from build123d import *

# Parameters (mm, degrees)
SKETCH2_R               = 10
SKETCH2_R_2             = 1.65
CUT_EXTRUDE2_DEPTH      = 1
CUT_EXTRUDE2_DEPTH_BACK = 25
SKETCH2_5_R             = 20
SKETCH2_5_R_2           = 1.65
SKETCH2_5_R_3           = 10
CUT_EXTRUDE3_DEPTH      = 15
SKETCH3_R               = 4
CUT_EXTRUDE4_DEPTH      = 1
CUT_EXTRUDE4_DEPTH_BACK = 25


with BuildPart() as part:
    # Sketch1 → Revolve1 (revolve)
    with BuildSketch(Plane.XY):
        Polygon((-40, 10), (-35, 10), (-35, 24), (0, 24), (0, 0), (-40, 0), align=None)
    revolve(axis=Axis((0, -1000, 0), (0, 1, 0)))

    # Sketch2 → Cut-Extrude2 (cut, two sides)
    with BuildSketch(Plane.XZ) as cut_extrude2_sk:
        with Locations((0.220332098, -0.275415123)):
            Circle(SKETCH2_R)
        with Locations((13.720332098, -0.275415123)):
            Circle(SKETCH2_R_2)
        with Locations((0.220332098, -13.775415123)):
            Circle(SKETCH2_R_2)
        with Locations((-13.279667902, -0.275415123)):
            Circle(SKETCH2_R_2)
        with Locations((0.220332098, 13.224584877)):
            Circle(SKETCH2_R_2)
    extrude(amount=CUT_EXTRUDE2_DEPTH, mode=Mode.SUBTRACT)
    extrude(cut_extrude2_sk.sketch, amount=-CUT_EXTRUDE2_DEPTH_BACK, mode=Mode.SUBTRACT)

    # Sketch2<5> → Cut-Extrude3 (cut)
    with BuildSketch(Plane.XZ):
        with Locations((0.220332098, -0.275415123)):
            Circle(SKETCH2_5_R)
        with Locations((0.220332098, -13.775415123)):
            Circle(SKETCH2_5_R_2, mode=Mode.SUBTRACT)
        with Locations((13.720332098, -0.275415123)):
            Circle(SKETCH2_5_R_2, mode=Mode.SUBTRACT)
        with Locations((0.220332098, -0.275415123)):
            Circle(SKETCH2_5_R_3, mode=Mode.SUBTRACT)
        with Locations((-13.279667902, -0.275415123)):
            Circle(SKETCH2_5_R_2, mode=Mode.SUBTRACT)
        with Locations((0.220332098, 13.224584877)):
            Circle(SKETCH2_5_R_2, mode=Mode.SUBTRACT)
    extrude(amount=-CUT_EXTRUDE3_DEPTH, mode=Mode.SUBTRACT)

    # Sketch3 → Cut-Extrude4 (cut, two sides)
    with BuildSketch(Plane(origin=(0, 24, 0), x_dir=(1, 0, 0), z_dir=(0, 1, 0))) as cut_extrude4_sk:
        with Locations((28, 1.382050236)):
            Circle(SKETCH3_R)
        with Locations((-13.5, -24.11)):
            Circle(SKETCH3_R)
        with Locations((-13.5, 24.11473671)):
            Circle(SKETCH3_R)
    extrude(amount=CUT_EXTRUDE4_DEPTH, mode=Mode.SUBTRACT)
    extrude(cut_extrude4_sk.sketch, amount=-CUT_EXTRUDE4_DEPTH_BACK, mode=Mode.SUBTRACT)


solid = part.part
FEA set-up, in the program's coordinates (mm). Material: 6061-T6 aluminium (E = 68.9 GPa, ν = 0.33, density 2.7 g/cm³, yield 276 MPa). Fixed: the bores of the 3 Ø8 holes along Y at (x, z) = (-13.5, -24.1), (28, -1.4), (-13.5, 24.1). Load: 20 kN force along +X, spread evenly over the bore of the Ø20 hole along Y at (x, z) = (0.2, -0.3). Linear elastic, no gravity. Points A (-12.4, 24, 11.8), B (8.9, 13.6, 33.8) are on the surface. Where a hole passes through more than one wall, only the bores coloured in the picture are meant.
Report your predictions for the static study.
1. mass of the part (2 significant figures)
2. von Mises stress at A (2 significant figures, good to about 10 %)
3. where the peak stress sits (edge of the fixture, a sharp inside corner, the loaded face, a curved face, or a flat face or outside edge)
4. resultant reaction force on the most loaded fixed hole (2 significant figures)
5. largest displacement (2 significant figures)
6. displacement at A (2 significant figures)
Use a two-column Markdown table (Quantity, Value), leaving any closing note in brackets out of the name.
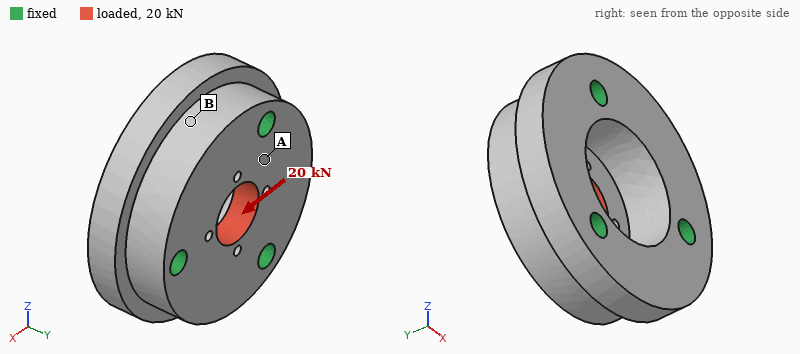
| Quantity | Value |
|---|---|
| mass of the part | 210 g |
| von Mises stress at A | 27 MPa |
| where the peak stress sits | a curved face |
| resultant reaction force on the most loaded fixed hole | 6.9 kN |
| largest displacement | 20 µm |
| displacement at A | 8.6 µm |
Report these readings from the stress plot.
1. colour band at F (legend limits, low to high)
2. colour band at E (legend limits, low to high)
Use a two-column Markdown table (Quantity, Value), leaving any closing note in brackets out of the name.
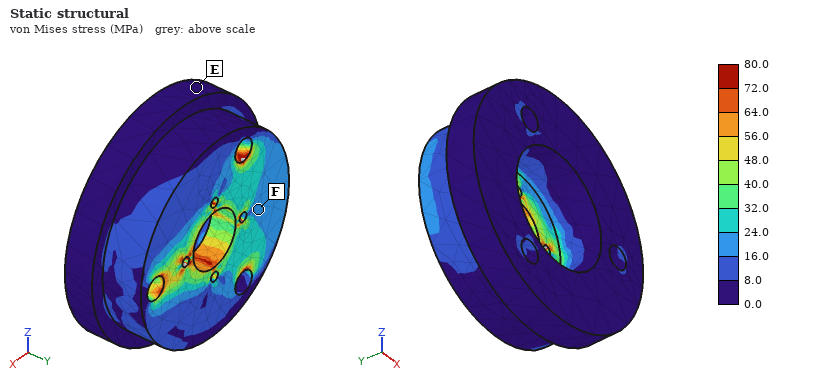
| Quantity | Value |
|---|---|
| colour band at F | 16.0 to 24.0 MPa |
| colour band at E | 0.0 to 8.0 MPa |
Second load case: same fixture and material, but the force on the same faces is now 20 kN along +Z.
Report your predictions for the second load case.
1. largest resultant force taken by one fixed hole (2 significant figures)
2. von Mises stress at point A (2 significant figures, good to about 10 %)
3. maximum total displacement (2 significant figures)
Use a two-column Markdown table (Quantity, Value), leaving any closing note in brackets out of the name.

| Quantity | Value |
|---|---|
| largest resultant force taken by one fixed hole | 7.0 kN |
| von Mises stress at point A | 30 MPa |
| maximum total displacement | 17 µm |
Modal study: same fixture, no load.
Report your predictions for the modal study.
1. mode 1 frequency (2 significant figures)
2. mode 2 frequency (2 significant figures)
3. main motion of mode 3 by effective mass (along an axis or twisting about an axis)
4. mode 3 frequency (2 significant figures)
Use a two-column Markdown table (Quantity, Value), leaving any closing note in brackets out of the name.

| Quantity | Value |
|---|---|
| mode 1 frequency | 18 kHz |
| mode 2 frequency | 18 kHz |
| main motion of mode 3 by effective mass | along Y |
| mode 3 frequency | 20 kHz |
